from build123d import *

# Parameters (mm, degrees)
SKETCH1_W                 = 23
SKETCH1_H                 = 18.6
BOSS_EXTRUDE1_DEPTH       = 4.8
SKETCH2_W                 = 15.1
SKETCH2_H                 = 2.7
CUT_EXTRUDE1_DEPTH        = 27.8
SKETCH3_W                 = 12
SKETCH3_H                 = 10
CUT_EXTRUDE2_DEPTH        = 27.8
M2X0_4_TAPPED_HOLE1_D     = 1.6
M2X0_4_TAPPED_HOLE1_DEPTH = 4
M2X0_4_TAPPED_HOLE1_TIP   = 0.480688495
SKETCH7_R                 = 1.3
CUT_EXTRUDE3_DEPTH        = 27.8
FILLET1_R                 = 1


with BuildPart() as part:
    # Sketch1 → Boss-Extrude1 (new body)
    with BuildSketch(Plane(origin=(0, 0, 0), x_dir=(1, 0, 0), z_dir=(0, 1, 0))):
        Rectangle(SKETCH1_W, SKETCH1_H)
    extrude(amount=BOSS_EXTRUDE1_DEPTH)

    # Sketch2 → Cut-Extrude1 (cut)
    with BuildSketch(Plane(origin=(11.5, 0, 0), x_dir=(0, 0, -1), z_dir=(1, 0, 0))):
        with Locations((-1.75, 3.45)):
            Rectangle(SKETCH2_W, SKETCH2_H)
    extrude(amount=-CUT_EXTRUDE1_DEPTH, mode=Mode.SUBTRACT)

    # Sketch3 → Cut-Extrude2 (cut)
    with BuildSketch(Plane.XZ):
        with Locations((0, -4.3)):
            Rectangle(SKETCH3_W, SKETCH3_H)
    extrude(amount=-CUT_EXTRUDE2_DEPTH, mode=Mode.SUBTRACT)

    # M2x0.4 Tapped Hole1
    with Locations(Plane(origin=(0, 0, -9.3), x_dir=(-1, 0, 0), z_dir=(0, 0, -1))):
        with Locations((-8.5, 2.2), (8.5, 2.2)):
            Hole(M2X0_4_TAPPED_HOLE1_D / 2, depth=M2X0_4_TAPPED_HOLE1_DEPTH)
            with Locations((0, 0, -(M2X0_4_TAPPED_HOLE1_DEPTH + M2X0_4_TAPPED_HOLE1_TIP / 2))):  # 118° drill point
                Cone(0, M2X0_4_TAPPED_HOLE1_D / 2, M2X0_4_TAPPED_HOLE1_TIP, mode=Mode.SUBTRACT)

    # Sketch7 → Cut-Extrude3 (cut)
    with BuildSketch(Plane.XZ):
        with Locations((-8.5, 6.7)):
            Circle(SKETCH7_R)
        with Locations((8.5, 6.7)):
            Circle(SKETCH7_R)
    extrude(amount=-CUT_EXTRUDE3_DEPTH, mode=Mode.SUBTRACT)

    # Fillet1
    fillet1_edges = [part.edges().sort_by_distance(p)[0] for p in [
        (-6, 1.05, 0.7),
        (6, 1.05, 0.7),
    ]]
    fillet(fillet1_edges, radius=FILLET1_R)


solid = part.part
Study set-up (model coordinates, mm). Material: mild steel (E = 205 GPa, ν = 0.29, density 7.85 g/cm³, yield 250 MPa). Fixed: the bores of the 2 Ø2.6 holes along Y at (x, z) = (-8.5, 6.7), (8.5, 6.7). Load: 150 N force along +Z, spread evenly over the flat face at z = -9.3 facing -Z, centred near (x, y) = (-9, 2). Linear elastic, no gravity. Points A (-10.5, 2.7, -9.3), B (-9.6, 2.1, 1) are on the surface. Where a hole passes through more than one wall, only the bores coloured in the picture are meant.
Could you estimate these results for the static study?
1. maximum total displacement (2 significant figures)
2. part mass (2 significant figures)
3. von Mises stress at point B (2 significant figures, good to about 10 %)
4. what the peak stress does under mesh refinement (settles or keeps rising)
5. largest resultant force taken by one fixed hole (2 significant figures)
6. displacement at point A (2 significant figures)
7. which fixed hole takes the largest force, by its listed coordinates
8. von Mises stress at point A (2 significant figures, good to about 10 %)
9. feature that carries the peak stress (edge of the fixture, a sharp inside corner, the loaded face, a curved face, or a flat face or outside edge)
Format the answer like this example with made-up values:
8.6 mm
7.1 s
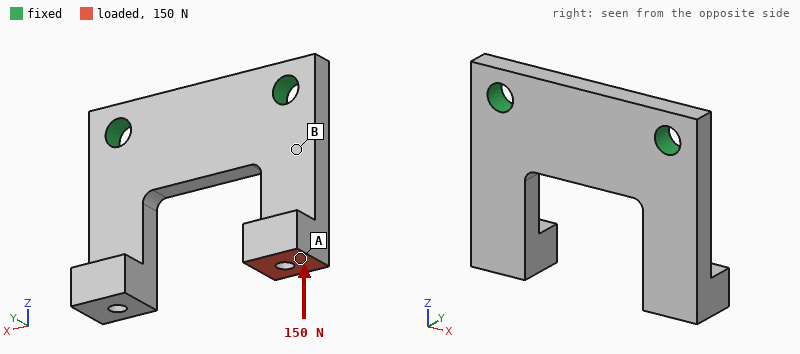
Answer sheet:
25 µm
5.6 g
57 MPa
keeps rising
150 N
23 µm
(-8.5, 6.7)
11 MPa
a sharp inside corner
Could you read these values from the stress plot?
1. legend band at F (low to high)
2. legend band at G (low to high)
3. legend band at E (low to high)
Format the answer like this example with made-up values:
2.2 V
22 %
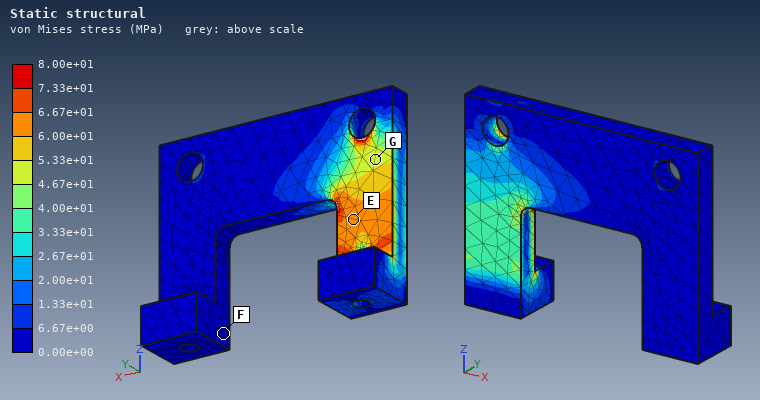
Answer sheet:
0.00e+00 to 6.67e+00 MPa
4.67e+01 to 5.33e+01 MPa
6.00e+01 to 6.67e+01 MPa
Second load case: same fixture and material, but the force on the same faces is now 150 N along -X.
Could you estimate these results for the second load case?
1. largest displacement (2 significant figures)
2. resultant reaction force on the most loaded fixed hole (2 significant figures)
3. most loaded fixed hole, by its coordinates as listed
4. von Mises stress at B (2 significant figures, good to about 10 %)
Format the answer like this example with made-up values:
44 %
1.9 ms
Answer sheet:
29 µm
180 N
(8.5, 6.7)
60 MPa
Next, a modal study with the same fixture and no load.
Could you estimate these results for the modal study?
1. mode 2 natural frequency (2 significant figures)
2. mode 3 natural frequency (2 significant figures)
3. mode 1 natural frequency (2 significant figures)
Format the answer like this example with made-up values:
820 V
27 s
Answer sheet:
6400 Hz
16 kHz
6200 Hz
